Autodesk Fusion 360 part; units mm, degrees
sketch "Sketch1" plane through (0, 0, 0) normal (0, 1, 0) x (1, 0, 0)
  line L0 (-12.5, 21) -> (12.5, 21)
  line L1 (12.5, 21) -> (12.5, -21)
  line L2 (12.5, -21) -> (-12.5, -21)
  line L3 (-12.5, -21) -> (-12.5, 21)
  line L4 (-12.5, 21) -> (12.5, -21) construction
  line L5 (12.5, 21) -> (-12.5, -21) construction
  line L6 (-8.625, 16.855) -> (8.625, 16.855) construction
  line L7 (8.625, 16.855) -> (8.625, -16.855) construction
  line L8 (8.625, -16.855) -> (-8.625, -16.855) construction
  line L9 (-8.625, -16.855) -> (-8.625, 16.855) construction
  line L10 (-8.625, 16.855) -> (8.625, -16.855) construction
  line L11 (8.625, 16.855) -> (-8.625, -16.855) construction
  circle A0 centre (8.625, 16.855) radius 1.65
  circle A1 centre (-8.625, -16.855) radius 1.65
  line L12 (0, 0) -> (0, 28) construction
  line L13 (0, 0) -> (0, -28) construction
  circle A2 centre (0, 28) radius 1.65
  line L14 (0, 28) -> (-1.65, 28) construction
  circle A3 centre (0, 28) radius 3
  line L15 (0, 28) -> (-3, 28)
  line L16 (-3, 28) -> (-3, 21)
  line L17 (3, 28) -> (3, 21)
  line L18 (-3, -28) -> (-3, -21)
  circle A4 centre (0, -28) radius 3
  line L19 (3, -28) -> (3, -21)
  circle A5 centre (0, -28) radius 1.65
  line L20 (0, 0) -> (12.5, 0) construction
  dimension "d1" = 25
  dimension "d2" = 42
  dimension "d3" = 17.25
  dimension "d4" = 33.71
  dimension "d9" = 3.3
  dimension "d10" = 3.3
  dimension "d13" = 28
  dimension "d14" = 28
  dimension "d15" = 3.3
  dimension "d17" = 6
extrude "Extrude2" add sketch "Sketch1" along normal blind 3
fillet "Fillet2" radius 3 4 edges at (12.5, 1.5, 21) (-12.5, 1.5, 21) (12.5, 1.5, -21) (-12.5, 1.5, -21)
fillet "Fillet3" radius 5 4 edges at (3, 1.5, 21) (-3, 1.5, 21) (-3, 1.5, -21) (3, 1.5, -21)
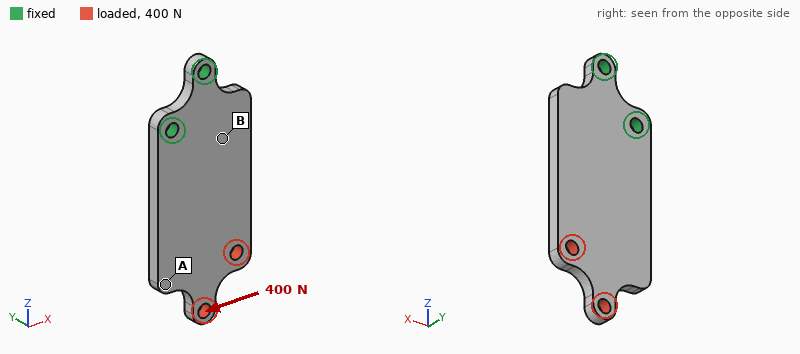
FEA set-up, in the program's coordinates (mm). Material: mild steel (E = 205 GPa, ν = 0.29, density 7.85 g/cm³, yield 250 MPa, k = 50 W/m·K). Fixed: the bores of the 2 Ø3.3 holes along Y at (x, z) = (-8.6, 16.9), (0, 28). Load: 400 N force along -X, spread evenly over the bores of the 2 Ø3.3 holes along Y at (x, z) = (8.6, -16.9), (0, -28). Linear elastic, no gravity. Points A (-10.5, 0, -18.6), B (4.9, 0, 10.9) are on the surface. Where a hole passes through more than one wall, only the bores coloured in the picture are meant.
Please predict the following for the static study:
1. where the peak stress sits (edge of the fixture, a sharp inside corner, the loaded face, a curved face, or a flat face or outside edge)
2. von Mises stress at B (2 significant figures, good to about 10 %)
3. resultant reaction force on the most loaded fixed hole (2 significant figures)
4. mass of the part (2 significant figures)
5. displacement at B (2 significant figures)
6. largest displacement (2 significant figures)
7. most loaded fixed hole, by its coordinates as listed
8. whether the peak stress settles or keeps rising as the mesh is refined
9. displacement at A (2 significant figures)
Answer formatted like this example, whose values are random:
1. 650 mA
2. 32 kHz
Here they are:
1. edge of the fixture
2. 28 MPa
3. 1.3 kN
4. 27 g
5. 6.5 µm
6. 40 µm
7. (-8.6, 16.9)
8. keeps rising
9. 26 µm
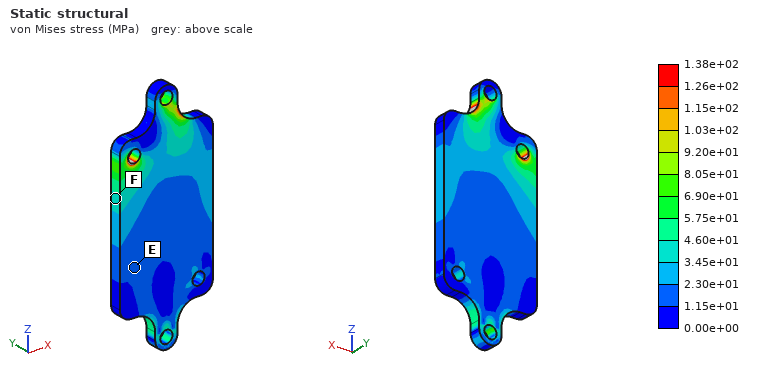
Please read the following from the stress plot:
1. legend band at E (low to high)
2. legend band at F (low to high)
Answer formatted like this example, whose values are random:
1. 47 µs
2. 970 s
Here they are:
1. 1.15e+01 to 2.30e+01 MPa
2. 3.45e+01 to 4.60e+01 MPa
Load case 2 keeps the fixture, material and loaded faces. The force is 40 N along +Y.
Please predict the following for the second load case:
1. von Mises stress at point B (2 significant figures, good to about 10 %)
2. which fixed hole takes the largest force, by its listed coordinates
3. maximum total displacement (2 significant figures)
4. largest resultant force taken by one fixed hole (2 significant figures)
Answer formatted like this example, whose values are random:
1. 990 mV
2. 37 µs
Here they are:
1. 29 MPa
2. (-8.6, 16.9)
3. 0.12 mm
4. 89 N
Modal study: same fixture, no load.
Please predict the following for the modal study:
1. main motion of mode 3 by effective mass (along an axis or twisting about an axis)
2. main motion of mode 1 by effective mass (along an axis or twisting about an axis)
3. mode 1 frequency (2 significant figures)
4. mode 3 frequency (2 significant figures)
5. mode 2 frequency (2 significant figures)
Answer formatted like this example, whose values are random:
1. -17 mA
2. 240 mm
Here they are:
1. along X
2. along Y
3. 1300 Hz
4. 6400 Hz
5. 4200 Hz
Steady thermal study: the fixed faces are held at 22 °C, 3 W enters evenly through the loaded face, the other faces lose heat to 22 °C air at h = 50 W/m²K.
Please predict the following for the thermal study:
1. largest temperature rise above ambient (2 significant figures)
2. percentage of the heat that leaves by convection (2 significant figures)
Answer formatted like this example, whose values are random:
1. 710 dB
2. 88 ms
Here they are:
1. 35 K
2. 49 %
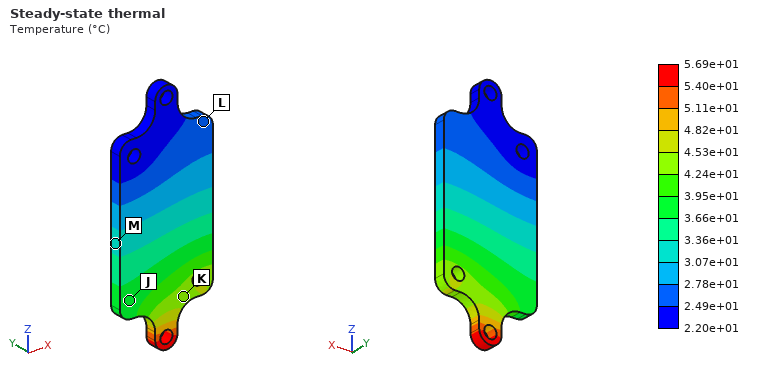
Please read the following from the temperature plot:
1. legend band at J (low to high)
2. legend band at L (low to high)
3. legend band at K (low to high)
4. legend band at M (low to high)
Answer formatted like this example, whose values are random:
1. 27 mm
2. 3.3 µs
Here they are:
1. 3.66e+01 to 3.95e+01 °C
2. 2.49e+01 to 2.78e+01 °C
3. 4.24e+01 to 4.53e+01 °C
4. 3.07e+01 to 3.36e+01 °C
